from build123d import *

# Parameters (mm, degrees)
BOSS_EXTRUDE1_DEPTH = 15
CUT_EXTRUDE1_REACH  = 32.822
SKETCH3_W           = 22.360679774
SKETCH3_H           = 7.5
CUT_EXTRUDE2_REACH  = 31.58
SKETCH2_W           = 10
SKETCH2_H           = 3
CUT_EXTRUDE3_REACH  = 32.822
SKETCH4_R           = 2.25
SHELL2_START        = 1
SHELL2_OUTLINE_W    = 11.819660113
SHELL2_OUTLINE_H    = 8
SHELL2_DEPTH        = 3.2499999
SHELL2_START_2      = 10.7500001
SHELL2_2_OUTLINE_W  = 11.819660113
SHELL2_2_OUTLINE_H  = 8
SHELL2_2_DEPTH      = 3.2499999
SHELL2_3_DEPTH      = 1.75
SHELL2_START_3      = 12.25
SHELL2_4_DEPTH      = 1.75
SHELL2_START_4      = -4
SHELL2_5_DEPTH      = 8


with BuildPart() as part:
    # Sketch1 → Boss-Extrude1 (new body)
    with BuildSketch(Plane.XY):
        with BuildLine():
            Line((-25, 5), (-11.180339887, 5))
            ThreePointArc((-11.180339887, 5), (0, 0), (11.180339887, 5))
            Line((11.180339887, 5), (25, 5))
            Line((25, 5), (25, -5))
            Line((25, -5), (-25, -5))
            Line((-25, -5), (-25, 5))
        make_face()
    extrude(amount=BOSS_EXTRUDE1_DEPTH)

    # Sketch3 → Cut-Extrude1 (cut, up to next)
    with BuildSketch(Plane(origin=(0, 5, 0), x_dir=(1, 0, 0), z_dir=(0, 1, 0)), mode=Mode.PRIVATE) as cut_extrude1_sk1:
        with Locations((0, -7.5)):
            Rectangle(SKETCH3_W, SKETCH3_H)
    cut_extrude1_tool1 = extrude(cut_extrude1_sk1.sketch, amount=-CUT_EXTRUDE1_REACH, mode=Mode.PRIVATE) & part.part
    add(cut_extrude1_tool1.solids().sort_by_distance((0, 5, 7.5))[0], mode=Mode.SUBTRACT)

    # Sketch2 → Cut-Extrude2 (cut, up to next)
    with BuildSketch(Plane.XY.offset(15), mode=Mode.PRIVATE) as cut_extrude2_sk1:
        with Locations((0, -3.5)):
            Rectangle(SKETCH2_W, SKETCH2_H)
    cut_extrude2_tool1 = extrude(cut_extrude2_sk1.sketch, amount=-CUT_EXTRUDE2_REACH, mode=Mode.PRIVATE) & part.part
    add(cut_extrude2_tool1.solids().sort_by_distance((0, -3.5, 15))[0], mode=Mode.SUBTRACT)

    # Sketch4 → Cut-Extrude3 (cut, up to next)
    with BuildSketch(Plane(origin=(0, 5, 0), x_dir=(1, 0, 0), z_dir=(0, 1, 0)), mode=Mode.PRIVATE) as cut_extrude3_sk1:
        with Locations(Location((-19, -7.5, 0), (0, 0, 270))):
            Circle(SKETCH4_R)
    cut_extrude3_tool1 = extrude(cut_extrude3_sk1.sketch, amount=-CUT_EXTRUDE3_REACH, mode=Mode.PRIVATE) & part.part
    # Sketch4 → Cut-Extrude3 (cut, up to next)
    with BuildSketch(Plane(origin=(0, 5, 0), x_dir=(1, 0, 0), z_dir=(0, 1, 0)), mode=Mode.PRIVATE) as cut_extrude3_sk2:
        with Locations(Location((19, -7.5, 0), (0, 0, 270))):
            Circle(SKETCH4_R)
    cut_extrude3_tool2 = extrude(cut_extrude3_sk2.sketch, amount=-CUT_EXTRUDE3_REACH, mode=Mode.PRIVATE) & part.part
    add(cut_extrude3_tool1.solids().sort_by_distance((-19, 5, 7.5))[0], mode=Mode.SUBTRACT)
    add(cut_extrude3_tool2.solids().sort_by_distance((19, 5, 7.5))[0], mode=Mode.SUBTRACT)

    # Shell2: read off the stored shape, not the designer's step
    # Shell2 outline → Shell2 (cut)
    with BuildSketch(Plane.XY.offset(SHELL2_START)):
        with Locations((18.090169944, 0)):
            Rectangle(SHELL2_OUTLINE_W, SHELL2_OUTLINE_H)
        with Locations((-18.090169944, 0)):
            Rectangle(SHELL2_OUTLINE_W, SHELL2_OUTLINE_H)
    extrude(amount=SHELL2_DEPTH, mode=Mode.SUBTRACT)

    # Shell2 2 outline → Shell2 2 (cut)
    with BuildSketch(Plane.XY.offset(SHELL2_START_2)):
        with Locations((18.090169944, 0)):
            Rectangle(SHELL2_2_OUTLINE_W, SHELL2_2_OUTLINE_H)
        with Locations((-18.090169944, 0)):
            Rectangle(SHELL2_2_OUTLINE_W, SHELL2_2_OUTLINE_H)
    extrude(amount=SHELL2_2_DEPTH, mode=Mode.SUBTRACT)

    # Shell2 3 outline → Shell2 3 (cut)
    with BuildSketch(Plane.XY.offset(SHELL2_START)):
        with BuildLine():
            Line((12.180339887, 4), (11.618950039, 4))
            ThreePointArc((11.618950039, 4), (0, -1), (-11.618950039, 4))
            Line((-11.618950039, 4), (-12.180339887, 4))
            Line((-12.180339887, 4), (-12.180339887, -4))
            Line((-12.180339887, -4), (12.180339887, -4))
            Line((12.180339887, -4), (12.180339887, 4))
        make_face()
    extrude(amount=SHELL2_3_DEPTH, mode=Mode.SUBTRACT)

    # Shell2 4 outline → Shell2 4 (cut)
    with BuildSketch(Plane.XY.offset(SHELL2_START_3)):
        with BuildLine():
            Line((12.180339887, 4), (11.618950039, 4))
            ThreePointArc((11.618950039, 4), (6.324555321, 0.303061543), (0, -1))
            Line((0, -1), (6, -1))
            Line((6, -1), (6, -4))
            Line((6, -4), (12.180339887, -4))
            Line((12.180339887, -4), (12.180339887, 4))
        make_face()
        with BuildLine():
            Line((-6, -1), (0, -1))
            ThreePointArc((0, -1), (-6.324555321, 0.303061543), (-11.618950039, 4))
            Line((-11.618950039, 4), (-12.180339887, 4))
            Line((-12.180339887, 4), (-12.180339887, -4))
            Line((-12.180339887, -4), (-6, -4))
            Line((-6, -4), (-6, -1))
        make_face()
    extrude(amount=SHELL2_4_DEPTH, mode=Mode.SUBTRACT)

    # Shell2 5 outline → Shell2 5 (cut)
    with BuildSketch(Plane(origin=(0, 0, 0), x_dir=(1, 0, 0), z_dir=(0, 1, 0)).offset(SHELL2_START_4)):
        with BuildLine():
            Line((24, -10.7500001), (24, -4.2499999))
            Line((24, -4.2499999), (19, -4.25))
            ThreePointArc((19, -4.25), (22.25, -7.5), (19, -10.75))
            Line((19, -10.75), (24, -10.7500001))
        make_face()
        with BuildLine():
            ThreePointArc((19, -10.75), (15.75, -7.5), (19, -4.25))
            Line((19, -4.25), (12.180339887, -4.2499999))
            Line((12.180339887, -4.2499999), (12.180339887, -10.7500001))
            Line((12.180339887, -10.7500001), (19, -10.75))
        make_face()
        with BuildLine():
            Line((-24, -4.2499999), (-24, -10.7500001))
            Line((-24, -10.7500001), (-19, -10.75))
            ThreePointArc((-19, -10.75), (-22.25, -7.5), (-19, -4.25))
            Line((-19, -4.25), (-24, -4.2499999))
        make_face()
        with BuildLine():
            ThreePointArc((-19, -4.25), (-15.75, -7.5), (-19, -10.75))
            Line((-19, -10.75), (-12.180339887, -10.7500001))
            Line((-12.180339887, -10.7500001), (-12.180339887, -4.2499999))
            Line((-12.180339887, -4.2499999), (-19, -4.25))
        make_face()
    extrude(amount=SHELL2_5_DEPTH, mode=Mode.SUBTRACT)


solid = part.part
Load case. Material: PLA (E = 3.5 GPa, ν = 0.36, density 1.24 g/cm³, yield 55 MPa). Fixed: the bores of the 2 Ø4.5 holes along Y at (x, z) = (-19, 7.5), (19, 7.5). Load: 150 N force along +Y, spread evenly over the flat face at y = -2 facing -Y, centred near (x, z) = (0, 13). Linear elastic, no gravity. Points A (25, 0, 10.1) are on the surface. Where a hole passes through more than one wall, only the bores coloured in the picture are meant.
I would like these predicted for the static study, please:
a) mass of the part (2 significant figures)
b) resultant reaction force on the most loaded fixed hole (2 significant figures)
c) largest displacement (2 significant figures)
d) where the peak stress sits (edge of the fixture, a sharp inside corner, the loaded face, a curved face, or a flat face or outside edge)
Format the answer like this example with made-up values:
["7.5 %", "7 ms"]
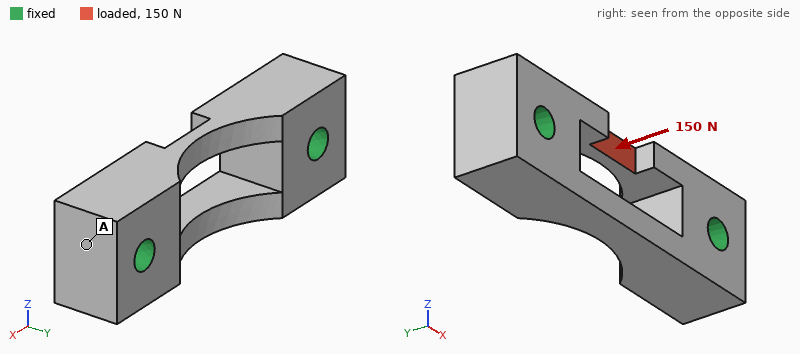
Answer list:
["3.2 g", "79 N", "0.31 mm", "a flat face or outside edge"]
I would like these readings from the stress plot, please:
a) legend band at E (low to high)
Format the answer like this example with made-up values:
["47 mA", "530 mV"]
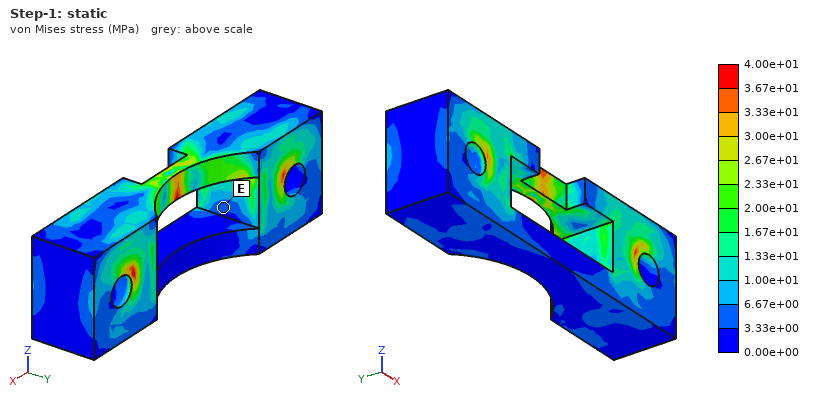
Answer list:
["3.33e+00 to 6.67e+00 MPa"]
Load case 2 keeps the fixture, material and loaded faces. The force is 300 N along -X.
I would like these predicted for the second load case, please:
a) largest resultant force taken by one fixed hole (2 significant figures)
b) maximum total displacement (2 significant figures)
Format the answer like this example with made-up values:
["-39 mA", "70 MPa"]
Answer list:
["150 N", "0.11 mm"]
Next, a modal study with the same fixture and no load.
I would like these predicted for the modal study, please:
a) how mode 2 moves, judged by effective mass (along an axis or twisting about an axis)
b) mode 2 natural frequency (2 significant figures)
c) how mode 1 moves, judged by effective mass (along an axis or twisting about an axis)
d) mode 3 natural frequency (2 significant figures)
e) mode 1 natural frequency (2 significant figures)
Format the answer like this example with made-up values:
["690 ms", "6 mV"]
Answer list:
["along Z", "6500 Hz", "along Y", "7800 Hz", "5400 Hz"]
